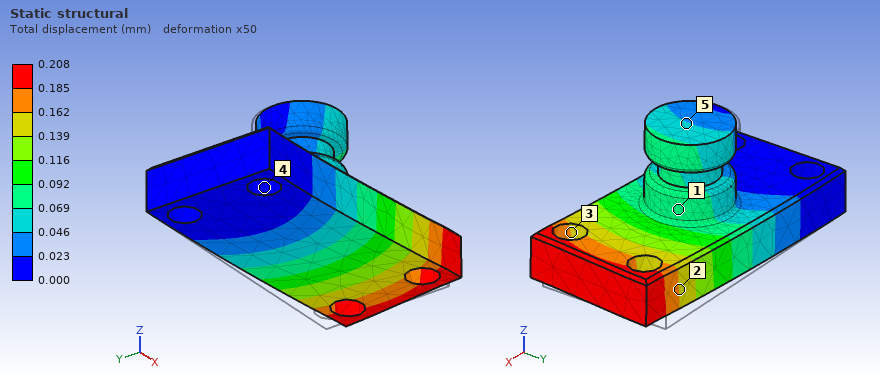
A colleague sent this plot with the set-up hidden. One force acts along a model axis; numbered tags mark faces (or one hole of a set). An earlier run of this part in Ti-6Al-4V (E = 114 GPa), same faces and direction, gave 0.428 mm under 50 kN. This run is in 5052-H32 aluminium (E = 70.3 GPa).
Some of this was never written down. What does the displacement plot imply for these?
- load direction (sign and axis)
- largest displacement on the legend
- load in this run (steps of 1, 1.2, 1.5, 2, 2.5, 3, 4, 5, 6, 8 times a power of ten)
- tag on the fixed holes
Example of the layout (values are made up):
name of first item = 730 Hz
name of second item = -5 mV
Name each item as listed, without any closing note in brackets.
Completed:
load direction = -Y
largest displacement on the legend = 0.208 mm
load in this run = 15 kN
tag on the fixed holes = 4
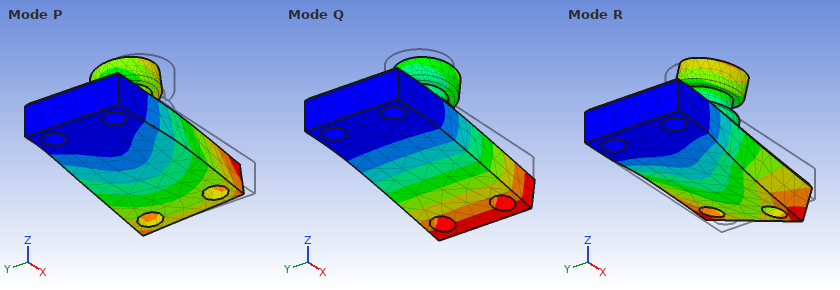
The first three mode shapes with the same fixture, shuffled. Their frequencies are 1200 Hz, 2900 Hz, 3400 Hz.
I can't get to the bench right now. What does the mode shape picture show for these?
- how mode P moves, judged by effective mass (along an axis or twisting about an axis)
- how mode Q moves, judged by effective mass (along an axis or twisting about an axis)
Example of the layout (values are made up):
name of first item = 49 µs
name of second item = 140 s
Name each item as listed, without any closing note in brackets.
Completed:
how mode P moves, judged by effective mass = along Y
how mode Q moves, judged by effective mass = along Z
